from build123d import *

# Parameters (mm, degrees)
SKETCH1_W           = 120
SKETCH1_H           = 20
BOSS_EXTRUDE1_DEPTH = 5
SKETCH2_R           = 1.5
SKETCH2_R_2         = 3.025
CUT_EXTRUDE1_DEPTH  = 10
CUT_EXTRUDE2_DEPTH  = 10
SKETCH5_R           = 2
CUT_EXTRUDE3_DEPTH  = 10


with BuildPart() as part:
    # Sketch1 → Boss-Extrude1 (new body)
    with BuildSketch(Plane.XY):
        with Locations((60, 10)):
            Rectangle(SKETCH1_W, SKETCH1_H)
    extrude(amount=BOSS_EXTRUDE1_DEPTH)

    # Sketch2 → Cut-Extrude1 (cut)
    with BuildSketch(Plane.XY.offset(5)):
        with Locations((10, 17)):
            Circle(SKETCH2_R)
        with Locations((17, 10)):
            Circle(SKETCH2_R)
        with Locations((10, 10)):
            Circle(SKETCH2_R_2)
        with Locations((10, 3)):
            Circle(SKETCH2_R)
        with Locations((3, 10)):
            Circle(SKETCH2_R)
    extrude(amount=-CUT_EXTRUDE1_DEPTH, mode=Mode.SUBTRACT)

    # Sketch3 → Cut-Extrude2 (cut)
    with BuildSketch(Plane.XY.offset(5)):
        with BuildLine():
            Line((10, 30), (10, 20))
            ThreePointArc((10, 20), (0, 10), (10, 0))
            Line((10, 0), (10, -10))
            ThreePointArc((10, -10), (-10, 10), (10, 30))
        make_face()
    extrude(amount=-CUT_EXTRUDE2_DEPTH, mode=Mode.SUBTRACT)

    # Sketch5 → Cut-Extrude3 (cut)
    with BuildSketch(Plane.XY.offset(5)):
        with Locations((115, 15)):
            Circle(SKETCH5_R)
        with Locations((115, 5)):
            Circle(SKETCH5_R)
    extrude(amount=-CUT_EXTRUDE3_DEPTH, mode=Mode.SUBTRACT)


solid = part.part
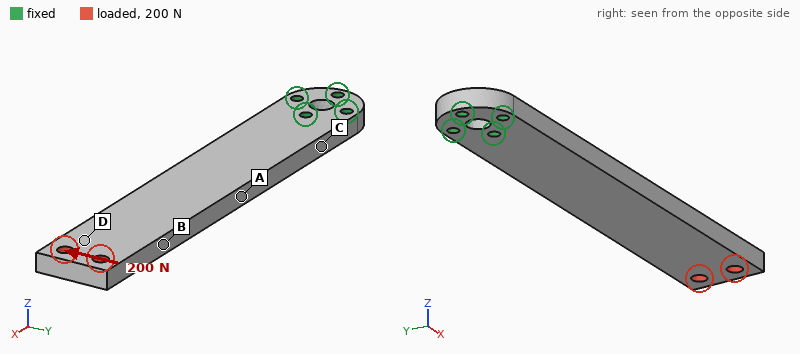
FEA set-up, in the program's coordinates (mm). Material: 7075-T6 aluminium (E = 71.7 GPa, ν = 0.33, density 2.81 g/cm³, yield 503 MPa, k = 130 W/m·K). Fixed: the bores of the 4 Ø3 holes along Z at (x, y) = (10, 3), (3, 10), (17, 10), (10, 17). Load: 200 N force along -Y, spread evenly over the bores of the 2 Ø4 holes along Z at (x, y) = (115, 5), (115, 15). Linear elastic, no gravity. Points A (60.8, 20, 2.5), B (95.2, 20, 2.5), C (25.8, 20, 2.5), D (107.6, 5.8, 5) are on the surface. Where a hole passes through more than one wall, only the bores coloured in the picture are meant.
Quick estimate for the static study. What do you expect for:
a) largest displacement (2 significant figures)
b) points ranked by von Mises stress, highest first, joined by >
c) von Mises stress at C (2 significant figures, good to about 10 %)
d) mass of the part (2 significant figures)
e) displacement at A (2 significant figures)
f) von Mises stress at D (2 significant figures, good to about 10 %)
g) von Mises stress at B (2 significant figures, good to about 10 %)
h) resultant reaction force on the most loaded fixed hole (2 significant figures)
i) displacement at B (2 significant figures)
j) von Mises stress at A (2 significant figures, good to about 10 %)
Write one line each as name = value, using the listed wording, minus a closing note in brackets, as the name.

largest displacement = 0.34 mm
points ranked by von Mises stress, highest first, joined by > = C > A > B > D
von Mises stress at C = 54 MPa
mass of the part = 32 g
displacement at A = 0.098 mm
von Mises stress at D = 5.0 MPa
von Mises stress at B = 12 MPa
resultant reaction force on the most loaded fixed hole = 1.1 kN
displacement at B = 0.23 mm
von Mises stress at A = 33 MPa
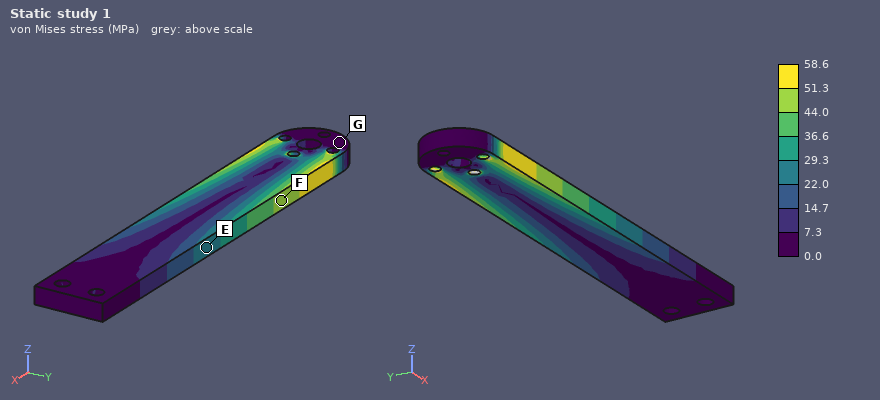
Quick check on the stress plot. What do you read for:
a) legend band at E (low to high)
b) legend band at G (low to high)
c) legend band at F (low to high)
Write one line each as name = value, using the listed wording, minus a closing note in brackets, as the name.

legend band at E = 22.0 to 29.3 MPa
legend band at G = 0.0 to 7.3 MPa
legend band at F = 44.0 to 51.3 MPa
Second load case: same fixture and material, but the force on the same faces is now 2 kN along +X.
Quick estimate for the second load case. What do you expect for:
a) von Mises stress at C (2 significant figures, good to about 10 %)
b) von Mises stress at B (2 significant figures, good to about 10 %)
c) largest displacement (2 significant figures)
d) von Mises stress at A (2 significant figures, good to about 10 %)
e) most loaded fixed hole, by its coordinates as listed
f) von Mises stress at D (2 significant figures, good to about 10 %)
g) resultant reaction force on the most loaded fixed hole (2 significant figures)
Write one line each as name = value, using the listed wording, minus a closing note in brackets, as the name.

von Mises stress at C = 17 MPa
von Mises stress at B = 20 MPa
largest displacement = 30 µm
von Mises stress at A = 20 MPa
most loaded fixed hole, by its coordinates as listed = (17, 10)
von Mises stress at D = 20 MPa
resultant reaction force on the most loaded fixed hole = 1.1 kN
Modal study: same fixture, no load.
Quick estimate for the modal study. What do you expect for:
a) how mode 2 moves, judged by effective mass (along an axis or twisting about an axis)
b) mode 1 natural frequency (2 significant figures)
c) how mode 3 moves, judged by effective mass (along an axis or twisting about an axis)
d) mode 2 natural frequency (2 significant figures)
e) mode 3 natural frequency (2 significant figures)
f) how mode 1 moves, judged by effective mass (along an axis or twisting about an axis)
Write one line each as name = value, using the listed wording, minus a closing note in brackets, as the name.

how mode 2 moves, judged by effective mass = along Y
mode 1 natural frequency = 390 Hz
how mode 3 moves, judged by effective mass = along Z
mode 2 natural frequency = 1400 Hz
mode 3 natural frequency = 2400 Hz
how mode 1 moves, judged by effective mass = along Z
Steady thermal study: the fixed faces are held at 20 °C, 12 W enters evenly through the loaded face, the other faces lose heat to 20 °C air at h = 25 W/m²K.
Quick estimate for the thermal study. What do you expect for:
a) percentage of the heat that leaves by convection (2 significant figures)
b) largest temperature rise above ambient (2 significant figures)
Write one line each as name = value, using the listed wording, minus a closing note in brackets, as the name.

percentage of the heat that leaves by convection = 37 %
largest temperature rise above ambient = 70 K
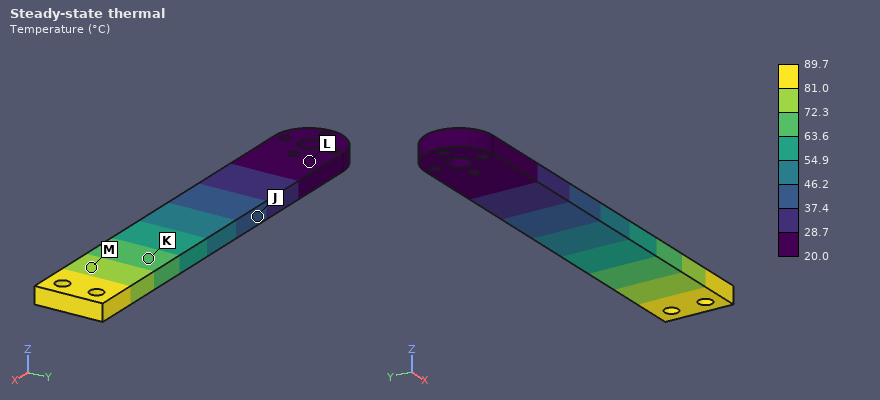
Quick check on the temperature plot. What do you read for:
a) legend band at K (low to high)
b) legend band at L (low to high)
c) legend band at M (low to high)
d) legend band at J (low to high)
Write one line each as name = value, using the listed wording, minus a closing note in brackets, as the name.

legend band at K = 63.6 to 72.3 °C
legend band at L = 20.0 to 28.7 °C
legend band at M = 72.3 to 81.0 °C
legend band at J = 37.4 to 46.2 °C
